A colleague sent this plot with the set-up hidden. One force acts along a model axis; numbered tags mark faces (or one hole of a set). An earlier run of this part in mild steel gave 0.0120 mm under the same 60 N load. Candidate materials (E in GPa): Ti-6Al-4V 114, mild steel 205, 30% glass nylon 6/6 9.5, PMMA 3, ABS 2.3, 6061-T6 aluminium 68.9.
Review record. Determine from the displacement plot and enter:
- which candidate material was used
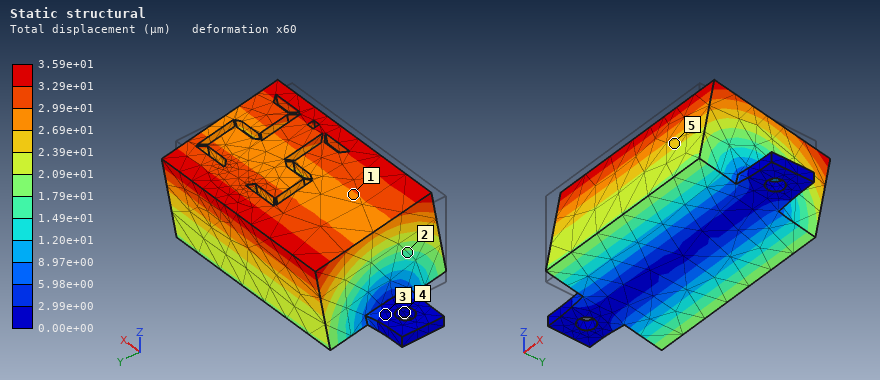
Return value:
6061-T6 aluminium
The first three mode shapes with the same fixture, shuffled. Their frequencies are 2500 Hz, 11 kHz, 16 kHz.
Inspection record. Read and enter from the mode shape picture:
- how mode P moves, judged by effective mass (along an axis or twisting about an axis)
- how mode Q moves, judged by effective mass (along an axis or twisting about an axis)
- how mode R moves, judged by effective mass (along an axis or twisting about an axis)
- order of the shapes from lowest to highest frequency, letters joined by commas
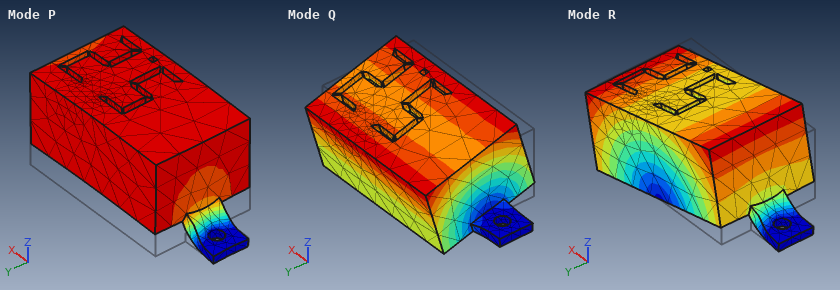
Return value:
along Z
along Y
along X
Q, P, R
